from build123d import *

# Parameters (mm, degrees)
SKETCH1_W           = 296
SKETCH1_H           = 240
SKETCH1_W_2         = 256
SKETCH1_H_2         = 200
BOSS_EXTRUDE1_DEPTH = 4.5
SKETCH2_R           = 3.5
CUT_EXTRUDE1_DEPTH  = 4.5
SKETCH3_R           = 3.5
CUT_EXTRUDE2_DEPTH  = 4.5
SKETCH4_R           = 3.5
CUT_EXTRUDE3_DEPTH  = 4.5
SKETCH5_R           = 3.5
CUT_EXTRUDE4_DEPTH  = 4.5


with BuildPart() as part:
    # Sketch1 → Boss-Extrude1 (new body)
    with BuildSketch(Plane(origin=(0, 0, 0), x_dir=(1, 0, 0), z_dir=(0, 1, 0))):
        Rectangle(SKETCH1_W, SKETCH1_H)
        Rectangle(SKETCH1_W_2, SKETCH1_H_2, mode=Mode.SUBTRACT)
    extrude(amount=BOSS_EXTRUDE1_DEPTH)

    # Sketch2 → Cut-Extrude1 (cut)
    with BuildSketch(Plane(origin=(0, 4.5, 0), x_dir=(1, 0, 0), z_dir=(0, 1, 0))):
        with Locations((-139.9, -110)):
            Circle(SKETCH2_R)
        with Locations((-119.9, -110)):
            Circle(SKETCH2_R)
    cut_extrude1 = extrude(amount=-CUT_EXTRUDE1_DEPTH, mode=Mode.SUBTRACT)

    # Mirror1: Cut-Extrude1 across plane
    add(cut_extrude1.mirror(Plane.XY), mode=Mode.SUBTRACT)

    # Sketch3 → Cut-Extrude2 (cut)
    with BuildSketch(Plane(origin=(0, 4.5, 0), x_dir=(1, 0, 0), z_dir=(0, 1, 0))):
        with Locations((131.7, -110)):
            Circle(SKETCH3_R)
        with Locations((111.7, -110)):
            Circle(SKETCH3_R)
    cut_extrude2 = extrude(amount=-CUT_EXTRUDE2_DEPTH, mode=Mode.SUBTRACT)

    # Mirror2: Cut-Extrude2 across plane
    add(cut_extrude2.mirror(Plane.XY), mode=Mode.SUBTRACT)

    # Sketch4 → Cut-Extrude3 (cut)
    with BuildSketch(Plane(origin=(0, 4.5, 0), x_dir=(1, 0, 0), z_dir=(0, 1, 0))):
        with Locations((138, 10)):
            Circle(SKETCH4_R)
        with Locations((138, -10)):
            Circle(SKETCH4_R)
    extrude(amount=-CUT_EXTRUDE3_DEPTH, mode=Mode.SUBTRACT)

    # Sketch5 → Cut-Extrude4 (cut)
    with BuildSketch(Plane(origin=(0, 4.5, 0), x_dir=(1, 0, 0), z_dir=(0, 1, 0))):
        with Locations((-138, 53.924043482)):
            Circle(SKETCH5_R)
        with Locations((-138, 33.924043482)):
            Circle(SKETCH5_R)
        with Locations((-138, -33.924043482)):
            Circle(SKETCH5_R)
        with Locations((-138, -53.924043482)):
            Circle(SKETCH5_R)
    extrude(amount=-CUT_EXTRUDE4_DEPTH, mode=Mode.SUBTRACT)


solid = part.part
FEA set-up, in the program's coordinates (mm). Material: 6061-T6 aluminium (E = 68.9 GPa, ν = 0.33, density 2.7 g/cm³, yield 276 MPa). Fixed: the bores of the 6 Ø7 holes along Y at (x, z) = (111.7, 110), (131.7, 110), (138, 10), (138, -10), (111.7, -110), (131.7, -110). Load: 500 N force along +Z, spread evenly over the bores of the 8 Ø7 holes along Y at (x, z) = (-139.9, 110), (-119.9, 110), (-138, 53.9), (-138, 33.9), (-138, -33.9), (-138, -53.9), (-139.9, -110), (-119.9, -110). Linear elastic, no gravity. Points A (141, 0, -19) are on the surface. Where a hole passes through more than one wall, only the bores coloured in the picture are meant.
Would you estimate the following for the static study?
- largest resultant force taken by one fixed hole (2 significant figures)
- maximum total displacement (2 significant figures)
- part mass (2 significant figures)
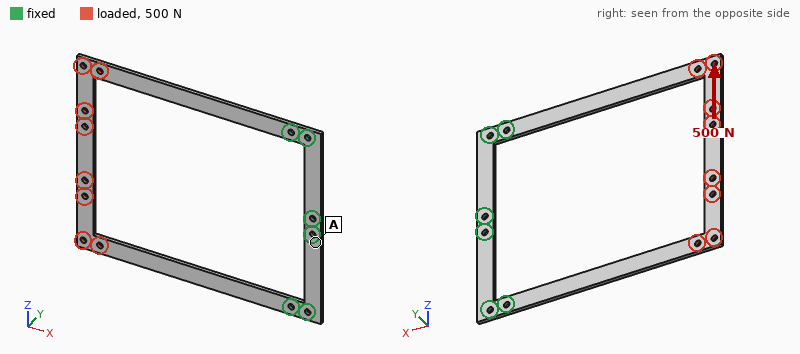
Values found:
980 N
2.3 mm
230 g
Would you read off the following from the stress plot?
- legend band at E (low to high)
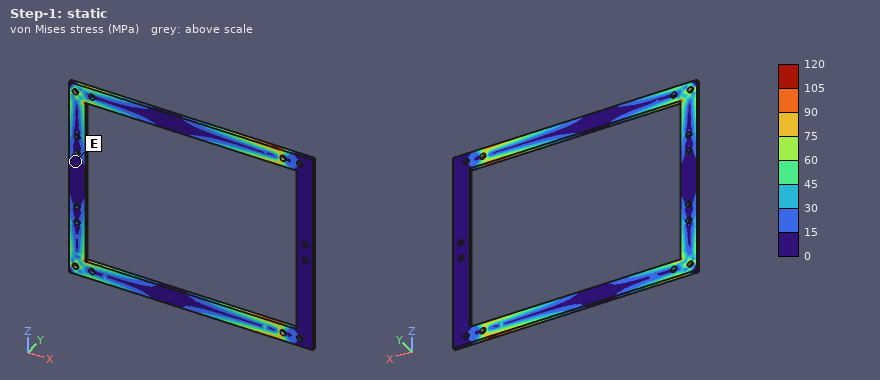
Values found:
0 to 15 MPa
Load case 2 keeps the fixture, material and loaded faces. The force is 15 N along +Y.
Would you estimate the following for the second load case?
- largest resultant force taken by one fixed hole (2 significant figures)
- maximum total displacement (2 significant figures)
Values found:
13 N
3.8 mm
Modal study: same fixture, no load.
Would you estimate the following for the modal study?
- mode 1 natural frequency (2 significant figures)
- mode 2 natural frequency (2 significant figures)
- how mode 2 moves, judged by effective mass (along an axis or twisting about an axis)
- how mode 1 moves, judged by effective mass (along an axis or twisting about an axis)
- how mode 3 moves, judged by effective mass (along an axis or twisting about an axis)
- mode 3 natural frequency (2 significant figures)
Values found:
36 Hz
89 Hz
twisting about X
along Y
along Z
250 Hz
